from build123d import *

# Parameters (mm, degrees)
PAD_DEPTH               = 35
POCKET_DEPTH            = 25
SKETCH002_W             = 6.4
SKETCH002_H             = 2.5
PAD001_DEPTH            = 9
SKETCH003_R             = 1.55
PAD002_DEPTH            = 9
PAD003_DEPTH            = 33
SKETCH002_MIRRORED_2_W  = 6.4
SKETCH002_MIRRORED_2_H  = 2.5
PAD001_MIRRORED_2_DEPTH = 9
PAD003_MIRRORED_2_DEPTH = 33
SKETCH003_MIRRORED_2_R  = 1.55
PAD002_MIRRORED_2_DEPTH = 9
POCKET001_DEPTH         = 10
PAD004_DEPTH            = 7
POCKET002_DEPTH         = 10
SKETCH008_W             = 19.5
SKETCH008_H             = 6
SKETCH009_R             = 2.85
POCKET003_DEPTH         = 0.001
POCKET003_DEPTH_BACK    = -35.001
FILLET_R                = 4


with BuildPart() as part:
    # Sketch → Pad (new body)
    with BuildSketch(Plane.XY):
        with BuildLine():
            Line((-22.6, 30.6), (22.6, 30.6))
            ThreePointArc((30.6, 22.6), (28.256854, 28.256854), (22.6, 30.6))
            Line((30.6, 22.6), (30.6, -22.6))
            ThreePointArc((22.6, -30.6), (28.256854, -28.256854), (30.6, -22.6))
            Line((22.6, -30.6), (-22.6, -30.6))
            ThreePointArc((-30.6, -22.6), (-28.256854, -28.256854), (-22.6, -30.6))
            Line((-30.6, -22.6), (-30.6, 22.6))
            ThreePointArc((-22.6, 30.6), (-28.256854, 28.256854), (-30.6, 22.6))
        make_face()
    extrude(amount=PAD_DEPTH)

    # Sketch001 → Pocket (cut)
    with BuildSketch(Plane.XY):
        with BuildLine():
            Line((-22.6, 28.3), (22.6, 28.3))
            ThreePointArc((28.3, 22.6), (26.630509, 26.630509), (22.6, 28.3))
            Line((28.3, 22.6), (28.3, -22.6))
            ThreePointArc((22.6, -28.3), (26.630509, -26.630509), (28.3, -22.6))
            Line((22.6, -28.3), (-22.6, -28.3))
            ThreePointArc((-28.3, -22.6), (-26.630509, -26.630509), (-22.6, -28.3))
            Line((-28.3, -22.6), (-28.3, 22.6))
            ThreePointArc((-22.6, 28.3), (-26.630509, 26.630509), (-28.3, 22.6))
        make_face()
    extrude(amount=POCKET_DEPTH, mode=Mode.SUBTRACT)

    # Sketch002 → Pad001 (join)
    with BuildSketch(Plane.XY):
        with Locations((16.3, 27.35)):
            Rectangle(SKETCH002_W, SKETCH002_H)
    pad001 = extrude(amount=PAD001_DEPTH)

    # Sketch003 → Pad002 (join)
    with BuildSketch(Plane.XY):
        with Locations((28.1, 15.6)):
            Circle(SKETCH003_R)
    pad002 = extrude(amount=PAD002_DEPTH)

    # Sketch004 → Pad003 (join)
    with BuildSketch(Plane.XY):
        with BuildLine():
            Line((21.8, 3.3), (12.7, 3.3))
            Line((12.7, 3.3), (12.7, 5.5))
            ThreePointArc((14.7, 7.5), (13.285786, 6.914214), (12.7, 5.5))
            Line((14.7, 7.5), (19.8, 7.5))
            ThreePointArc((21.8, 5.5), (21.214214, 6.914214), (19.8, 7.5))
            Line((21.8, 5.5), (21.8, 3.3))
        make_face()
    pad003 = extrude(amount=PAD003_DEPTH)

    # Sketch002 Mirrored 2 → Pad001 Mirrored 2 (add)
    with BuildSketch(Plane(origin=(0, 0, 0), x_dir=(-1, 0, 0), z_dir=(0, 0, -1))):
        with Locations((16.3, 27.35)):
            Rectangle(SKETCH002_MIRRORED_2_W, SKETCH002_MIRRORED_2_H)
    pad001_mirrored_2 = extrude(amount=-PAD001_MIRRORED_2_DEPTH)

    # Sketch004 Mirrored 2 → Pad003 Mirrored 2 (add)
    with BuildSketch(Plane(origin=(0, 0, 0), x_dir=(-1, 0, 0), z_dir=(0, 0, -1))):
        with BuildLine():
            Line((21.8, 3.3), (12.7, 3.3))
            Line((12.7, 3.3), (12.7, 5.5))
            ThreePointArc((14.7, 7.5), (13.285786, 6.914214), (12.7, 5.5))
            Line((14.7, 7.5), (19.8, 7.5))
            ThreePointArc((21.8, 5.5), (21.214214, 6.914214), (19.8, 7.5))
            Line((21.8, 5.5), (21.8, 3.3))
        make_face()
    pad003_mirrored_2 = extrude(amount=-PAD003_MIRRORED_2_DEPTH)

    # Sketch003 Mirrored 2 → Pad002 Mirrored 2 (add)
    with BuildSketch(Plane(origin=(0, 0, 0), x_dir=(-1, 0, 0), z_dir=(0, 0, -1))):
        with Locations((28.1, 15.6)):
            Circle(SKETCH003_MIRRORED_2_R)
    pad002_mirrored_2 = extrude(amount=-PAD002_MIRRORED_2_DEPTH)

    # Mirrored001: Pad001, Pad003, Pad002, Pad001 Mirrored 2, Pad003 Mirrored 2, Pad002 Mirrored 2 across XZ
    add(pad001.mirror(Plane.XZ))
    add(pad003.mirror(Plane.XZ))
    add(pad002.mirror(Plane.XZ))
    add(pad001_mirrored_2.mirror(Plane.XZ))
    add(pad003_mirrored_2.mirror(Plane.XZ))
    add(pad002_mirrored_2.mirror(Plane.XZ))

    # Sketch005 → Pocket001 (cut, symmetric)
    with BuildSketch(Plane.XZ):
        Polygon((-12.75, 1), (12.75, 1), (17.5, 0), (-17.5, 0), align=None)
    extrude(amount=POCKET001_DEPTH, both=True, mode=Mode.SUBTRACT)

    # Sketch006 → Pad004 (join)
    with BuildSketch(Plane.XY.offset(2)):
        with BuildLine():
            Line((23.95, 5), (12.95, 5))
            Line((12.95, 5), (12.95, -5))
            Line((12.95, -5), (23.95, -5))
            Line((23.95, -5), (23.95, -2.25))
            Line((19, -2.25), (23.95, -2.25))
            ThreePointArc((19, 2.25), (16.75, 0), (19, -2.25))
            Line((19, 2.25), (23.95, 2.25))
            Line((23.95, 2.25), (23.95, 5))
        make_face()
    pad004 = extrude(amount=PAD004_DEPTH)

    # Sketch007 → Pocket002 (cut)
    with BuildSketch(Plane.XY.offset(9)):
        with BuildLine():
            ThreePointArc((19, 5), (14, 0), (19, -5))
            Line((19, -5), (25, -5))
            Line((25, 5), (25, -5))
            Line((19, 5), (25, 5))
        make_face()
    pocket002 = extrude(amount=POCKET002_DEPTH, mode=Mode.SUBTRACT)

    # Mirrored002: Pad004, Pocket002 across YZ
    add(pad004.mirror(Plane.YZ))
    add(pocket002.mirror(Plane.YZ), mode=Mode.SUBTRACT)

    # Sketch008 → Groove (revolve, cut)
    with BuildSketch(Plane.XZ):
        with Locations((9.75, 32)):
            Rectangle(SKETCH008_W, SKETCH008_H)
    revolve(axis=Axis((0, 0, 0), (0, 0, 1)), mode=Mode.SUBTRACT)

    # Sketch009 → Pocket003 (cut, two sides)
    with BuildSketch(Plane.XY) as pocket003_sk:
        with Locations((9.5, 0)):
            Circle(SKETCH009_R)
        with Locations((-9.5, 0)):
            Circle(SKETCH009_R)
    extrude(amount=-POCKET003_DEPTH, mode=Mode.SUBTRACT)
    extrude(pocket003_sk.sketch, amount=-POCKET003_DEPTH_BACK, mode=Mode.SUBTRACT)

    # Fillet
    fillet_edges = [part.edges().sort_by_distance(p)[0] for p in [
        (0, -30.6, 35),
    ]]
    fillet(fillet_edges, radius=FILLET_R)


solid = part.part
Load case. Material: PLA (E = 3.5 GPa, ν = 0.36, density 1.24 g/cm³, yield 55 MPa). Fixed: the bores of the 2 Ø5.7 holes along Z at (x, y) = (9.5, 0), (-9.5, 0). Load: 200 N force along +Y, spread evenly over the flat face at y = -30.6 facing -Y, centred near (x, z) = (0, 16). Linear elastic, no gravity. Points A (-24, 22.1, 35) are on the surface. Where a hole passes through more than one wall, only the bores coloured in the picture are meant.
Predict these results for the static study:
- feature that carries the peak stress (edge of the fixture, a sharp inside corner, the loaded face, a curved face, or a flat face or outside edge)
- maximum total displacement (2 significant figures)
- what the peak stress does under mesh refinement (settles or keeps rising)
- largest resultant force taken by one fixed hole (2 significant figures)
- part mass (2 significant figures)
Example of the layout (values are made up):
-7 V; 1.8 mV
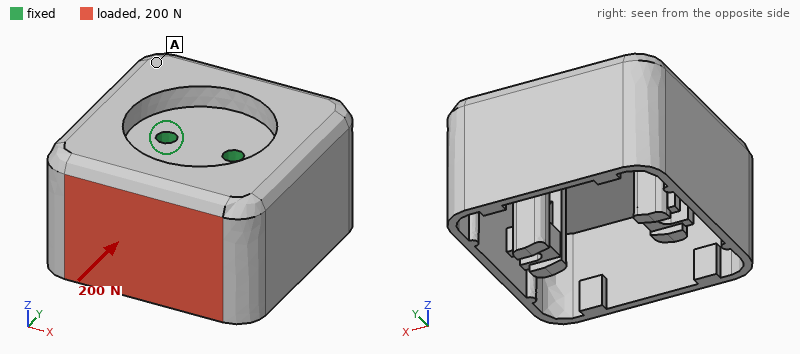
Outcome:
edge of the fixture; 1.0 mm; keeps rising; 100 N; 57 g
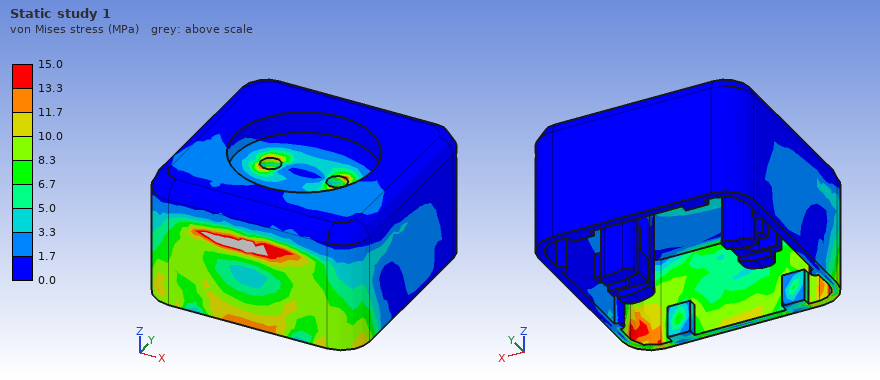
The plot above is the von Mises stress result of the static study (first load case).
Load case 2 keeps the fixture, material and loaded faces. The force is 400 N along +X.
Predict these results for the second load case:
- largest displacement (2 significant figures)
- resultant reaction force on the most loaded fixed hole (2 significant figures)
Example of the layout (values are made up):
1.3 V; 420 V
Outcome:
0.47 mm; 570 N
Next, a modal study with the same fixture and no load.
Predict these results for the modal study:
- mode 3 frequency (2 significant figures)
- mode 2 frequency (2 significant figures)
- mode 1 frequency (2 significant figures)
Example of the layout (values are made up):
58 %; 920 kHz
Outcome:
1200 Hz; 940 Hz; 570 Hz
